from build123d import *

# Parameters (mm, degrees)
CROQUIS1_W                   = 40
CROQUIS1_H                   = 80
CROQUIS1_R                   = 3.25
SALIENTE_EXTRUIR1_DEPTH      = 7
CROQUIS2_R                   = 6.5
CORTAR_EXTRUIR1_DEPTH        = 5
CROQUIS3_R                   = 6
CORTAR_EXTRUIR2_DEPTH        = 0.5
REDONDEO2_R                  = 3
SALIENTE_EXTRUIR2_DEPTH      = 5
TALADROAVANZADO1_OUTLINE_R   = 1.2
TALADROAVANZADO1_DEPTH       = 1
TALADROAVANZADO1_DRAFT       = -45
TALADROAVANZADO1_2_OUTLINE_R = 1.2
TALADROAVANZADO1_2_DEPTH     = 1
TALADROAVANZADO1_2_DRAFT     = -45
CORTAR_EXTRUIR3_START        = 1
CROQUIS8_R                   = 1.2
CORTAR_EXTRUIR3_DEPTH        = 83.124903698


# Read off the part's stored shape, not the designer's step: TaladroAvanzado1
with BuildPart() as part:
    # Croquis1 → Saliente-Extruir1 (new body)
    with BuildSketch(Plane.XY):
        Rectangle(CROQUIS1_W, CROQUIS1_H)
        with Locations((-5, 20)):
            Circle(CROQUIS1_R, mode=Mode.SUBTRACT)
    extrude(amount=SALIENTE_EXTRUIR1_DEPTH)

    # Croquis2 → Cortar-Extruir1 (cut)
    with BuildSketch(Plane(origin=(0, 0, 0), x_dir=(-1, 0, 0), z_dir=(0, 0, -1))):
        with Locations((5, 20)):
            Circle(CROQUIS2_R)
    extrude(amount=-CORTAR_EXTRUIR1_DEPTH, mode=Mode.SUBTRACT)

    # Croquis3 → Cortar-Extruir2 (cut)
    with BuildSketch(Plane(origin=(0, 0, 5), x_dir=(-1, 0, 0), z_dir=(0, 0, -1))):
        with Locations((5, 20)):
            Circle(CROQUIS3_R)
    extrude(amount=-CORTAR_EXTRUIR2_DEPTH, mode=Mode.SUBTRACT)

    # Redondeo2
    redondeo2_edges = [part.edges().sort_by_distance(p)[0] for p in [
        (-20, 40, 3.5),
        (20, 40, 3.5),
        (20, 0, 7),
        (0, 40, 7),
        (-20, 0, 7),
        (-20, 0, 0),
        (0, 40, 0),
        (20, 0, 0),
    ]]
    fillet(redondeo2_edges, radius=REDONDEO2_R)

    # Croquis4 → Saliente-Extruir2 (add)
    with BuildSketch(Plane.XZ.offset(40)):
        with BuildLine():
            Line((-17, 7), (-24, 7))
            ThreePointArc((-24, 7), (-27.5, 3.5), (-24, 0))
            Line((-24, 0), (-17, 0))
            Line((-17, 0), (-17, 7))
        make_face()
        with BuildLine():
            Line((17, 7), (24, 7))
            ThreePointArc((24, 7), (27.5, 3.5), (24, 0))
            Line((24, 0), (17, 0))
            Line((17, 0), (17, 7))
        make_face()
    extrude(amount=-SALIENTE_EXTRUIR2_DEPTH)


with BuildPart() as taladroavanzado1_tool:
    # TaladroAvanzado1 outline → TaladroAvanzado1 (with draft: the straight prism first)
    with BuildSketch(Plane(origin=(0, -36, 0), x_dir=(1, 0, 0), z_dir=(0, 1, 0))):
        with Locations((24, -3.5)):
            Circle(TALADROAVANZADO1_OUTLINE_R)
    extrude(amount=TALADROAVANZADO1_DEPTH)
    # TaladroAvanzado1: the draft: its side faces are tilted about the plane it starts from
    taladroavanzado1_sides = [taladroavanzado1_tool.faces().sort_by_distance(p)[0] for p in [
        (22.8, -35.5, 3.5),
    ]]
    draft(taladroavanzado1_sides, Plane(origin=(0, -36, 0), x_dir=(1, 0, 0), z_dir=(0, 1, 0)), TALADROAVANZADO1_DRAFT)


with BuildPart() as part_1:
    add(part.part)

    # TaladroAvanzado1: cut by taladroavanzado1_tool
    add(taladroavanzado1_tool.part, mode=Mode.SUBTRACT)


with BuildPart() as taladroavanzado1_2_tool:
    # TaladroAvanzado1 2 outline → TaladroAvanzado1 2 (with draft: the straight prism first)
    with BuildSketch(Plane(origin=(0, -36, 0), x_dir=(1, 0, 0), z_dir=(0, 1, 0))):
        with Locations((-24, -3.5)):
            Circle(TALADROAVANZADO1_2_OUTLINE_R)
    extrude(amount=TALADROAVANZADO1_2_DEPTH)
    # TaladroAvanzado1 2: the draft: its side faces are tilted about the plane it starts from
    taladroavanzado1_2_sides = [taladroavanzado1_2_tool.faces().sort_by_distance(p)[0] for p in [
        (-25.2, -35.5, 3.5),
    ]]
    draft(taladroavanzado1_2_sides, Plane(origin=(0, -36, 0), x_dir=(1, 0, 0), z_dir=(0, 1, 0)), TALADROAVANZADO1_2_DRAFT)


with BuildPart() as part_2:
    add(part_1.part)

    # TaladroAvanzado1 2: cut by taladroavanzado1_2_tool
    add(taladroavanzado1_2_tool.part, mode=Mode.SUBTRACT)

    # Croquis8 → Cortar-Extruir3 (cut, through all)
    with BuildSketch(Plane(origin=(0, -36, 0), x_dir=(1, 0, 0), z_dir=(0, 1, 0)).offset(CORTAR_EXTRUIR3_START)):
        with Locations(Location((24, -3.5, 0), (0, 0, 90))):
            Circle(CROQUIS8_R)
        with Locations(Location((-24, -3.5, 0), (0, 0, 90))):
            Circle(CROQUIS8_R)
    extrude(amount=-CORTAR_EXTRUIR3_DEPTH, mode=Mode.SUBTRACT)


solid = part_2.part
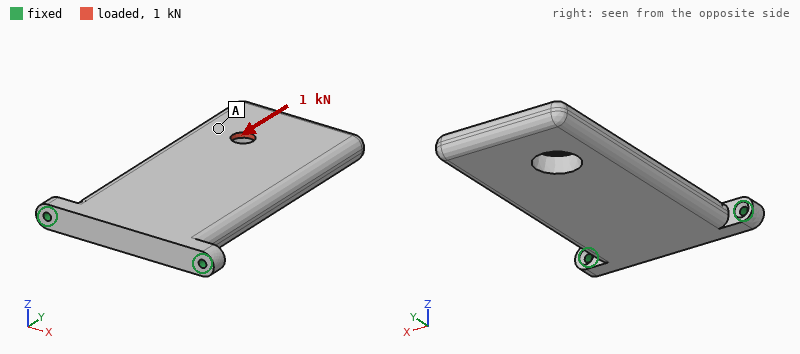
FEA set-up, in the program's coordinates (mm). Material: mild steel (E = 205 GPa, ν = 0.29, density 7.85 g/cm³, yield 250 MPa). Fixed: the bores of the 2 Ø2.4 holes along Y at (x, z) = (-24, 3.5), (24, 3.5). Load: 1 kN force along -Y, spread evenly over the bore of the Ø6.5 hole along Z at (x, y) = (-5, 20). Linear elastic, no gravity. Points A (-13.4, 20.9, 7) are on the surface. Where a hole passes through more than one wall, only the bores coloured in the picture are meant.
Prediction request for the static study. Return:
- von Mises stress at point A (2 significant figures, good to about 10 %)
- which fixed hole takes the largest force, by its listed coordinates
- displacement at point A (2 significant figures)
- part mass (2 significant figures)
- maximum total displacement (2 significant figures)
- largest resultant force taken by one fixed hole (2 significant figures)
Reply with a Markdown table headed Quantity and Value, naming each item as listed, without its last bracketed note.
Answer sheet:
| Quantity | Value |
|---|---|
| von Mises stress at point A | 9.6 MPa |
| which fixed hole takes the largest force, by its listed coordinates | (-24, 3.5) |
| displacement at point A | 66 µm |
| part mass | 170 g |
| maximum total displacement | 94 µm |
| largest resultant force taken by one fixed hole | 680 N |
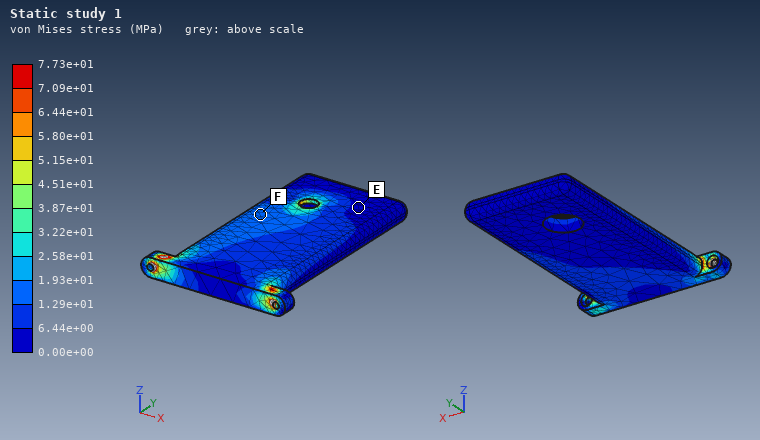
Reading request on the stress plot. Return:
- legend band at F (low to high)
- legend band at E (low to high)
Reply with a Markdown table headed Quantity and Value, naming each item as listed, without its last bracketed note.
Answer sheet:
| Quantity | Value |
|---|---|
| legend band at F | 1.29e+01 to 1.93e+01 MPa |
| legend band at E | 0.00e+00 to 6.44e+00 MPa |
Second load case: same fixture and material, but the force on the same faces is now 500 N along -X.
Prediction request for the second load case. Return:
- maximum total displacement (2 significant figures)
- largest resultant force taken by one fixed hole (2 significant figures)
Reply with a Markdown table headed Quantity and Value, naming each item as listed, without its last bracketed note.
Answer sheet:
| Quantity | Value |
|---|---|
| maximum total displacement | 20 µm |
| largest resultant force taken by one fixed hole | 720 N |
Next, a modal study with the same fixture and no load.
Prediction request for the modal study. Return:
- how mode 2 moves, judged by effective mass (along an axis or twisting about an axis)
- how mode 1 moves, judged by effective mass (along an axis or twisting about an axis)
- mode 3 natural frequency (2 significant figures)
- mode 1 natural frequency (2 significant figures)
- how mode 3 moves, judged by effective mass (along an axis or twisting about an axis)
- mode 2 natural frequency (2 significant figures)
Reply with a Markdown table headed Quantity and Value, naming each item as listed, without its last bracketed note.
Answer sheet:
| Quantity | Value |
|---|---|
| how mode 2 moves, judged by effective mass | along X |
| how mode 1 moves, judged by effective mass | along Z |
| mode 3 natural frequency | 3500 Hz |
| mode 1 natural frequency | 480 Hz |
| how mode 3 moves, judged by effective mass | twisting about Y |
| mode 2 natural frequency | 3100 Hz |
